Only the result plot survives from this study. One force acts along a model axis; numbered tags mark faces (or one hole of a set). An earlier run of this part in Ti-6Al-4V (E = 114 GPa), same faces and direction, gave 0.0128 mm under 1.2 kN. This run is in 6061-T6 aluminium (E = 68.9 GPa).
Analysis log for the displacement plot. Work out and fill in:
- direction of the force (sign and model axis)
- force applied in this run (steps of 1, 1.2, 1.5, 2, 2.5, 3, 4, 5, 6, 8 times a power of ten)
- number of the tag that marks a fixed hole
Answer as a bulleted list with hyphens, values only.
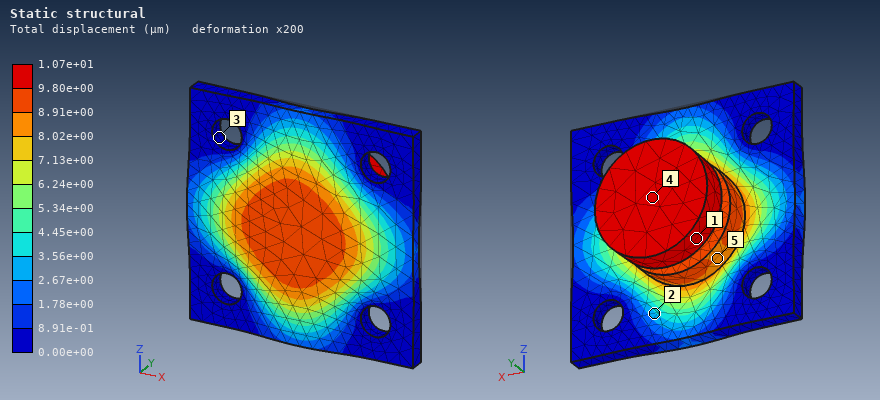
- -Y
- 600 N
- 3
